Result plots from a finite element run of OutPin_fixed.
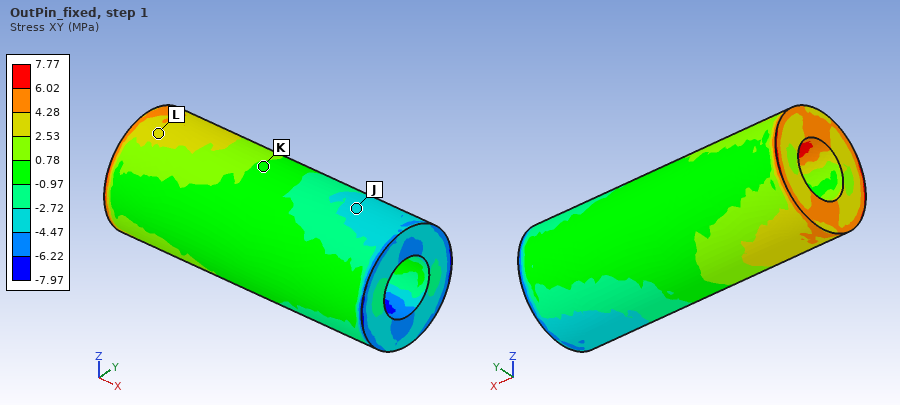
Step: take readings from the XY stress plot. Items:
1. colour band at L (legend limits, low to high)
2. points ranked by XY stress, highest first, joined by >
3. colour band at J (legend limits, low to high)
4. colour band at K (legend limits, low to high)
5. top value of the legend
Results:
2.53 to 4.28 MPa
L > K > J
-4.47 to -2.72 MPa
-0.97 to 0.78 MPa
7.77 MPa
